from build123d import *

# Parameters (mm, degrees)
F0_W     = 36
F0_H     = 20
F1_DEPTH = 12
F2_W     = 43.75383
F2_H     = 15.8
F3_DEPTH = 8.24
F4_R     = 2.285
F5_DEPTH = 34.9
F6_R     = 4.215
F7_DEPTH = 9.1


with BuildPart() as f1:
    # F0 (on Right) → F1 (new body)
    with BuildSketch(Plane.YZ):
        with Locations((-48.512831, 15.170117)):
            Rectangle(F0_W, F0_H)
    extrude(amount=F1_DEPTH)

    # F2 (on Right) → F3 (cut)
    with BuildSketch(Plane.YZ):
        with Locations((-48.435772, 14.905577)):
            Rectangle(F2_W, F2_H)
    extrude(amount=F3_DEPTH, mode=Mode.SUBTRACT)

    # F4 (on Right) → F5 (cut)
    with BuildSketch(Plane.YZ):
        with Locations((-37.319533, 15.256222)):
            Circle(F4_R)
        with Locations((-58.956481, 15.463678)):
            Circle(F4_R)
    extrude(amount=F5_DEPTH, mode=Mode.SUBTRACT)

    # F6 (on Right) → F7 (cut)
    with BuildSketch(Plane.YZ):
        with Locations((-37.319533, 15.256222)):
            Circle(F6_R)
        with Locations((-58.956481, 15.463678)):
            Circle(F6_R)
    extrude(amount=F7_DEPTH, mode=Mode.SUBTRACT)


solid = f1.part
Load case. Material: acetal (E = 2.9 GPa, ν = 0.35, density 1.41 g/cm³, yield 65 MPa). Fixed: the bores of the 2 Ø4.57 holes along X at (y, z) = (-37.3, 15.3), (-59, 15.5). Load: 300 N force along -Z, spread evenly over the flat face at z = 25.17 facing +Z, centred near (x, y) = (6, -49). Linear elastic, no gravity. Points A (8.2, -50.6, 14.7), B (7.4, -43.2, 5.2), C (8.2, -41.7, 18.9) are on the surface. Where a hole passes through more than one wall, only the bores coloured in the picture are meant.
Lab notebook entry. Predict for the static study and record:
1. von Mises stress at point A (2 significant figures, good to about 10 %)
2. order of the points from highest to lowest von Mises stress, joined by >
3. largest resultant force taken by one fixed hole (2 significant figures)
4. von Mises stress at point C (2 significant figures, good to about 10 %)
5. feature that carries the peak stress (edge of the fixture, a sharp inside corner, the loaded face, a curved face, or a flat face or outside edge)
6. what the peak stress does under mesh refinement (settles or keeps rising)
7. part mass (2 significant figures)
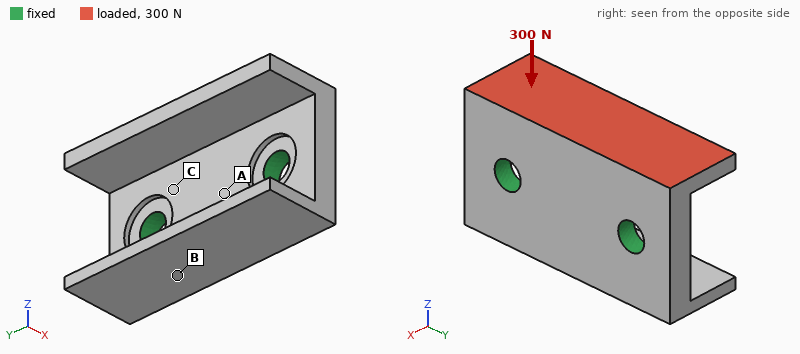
7.4 MPa
C > A > B
150 N
15 MPa
edge of the fixture
keeps rising
5.3 g
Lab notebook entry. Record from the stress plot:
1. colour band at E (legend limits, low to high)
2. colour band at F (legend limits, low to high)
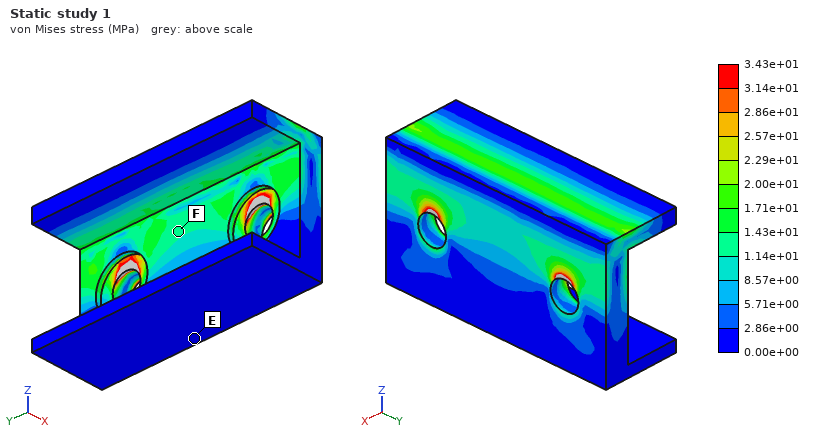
0.00e+00 to 2.86e+00 MPa
1.14e+01 to 1.43e+01 MPa
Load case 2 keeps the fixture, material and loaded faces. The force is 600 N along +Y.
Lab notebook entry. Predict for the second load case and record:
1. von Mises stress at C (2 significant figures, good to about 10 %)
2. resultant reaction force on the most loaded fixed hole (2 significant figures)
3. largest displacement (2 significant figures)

15 MPa
400 N
0.22 mm
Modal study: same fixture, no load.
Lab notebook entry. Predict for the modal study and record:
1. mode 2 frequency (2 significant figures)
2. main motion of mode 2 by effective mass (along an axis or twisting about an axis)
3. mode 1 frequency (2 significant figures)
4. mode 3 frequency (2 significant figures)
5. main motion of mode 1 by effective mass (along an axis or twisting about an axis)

3700 Hz
along X
3100 Hz
4100 Hz
along Z
